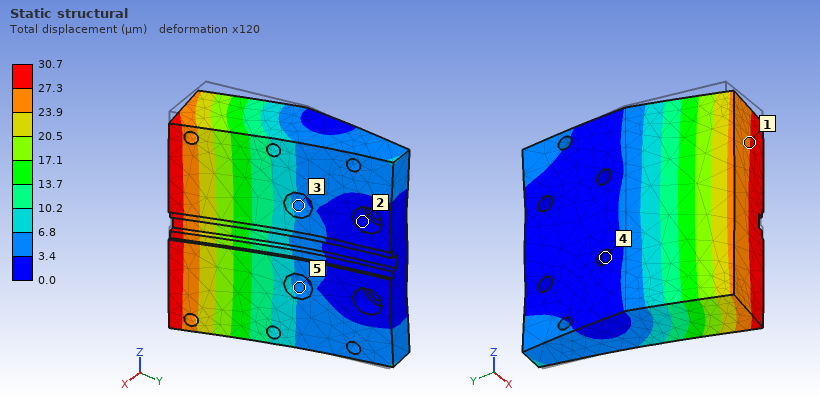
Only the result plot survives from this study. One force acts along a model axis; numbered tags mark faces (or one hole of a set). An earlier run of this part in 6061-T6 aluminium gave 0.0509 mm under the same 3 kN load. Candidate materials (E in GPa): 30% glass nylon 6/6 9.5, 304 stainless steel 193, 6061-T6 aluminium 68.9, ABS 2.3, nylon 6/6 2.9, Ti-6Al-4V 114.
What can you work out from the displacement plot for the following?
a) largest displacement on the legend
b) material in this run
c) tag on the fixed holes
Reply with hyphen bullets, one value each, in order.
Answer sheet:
- 30.7 µm
- Ti-6Al-4V
- 4
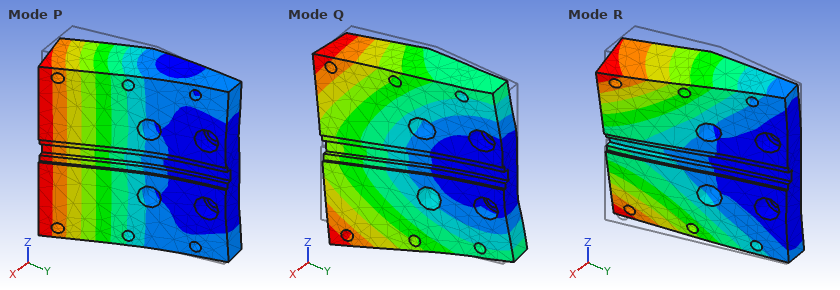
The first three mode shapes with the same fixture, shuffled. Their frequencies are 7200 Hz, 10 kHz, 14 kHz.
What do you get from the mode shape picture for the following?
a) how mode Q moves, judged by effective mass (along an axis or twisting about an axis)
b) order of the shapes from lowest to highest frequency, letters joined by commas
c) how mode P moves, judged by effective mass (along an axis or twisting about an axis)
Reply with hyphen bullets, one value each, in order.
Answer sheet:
- along Z
- P, R, Q
- along X
